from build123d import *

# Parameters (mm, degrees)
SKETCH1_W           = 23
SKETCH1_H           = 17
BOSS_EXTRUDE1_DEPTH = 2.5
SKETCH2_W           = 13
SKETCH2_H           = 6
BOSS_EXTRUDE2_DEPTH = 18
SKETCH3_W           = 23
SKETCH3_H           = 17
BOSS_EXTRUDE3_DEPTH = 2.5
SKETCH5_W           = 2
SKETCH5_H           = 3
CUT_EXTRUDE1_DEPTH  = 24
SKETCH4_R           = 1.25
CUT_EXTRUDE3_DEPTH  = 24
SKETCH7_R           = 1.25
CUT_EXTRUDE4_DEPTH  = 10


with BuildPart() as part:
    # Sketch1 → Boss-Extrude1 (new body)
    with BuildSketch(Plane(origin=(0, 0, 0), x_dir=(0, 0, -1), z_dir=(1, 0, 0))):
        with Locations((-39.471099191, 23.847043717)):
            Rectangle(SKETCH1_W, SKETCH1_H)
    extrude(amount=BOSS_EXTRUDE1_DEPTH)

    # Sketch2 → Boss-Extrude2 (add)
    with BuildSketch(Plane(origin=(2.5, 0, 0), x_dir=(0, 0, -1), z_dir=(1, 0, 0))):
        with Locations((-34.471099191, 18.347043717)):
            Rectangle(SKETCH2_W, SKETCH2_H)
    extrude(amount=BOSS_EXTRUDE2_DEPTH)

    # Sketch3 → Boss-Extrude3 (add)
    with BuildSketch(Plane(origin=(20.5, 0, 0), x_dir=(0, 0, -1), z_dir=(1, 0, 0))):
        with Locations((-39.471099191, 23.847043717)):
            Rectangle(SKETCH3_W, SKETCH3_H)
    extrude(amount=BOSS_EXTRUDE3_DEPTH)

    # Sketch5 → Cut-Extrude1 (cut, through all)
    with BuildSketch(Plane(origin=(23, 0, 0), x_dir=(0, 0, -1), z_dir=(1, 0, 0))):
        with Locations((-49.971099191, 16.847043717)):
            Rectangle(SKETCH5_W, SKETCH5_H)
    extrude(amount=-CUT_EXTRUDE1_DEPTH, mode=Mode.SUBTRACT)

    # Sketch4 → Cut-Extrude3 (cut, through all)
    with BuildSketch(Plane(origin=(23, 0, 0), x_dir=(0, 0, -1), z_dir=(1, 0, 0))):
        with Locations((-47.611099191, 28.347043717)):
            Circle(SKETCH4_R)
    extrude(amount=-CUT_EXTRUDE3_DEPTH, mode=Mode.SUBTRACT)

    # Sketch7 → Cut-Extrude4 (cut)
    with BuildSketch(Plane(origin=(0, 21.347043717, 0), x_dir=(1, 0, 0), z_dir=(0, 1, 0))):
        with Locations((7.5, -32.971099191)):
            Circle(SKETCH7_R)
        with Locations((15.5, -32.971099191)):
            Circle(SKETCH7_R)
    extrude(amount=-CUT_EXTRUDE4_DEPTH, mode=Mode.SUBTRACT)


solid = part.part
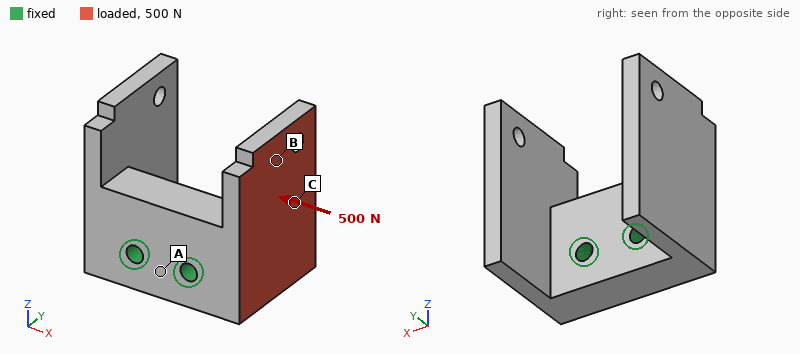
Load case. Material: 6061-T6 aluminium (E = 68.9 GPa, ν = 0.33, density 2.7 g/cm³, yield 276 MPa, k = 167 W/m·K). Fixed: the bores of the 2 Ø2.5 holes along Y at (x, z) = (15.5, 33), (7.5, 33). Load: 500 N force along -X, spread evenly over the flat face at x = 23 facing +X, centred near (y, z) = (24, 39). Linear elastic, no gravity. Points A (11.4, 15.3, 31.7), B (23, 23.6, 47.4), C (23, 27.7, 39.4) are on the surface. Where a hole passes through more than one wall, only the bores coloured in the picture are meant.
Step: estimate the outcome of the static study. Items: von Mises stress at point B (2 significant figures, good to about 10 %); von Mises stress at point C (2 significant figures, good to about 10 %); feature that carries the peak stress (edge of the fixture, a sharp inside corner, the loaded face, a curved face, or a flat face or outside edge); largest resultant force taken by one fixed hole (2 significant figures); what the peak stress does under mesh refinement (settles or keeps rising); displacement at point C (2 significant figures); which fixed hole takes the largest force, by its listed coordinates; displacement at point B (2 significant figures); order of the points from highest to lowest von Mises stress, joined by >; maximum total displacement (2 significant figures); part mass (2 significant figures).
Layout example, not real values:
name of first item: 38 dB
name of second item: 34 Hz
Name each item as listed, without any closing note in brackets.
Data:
von Mises stress at point B: 20 MPa
von Mises stress at point C: 32 MPa
feature that carries the peak stress: a sharp inside corner
largest resultant force taken by one fixed hole: 430 N
what the peak stress does under mesh refinement: keeps rising
displacement at point C: 0.047 mm
which fixed hole takes the largest force, by its listed coordinates: (15.5, 33)
displacement at point B: 0.055 mm
order of the points from highest to lowest von Mises stress, joined by >: C > B > A
maximum total displacement: 0.13 mm
part mass: 8.8 g
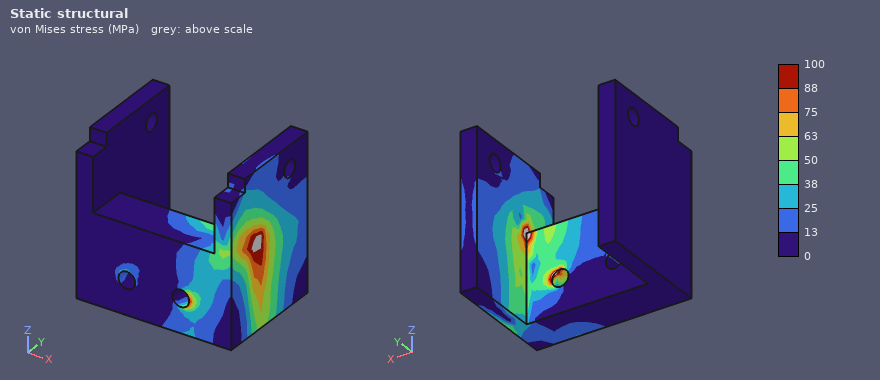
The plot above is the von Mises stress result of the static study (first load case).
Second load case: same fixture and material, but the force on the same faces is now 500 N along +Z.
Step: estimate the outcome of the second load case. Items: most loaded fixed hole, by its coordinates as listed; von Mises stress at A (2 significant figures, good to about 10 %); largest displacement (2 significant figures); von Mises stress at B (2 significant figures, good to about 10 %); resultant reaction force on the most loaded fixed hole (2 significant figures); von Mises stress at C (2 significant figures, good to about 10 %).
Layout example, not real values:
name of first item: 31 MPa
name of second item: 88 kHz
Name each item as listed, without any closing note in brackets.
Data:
most loaded fixed hole, by its coordinates as listed: (15.5, 33)
von Mises stress at A: 13 MPa
largest displacement: 40 µm
von Mises stress at B: 7.4 MPa
resultant reaction force on the most loaded fixed hole: 800 N
von Mises stress at C: 18 MPa
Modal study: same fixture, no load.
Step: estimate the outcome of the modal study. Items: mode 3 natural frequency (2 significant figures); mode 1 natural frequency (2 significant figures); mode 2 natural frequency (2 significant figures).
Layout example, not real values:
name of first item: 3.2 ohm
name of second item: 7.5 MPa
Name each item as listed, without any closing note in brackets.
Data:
mode 3 natural frequency: 12 kHz
mode 1 natural frequency: 8700 Hz
mode 2 natural frequency: 8900 Hz
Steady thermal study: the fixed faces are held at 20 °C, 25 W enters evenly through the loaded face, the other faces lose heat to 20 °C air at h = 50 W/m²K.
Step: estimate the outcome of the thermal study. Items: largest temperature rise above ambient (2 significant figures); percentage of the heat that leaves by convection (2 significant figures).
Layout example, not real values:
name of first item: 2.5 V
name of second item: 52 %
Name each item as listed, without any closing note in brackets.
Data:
largest temperature rise above ambient: 35 K
percentage of the heat that leaves by convection: 3.2 %
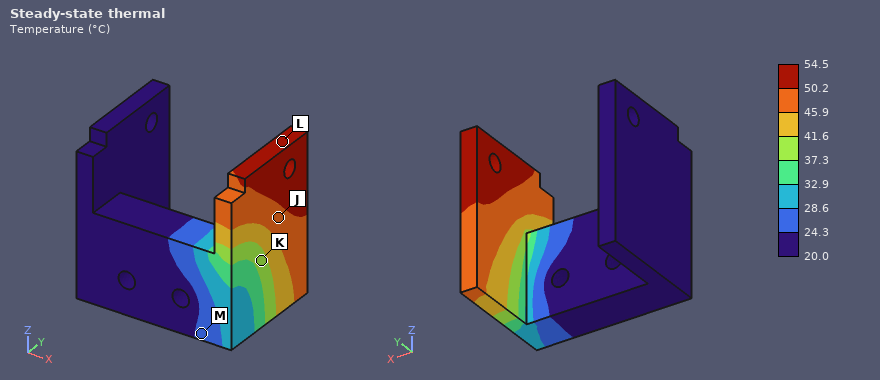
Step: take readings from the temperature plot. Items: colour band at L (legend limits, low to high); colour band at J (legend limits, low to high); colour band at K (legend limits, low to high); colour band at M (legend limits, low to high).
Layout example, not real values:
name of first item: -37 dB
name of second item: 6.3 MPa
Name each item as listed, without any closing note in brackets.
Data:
colour band at L: 50.2 to 54.5 °C
colour band at J: 45.9 to 50.2 °C
colour band at K: 37.3 to 41.6 °C
colour band at M: 24.3 to 28.6 °C
